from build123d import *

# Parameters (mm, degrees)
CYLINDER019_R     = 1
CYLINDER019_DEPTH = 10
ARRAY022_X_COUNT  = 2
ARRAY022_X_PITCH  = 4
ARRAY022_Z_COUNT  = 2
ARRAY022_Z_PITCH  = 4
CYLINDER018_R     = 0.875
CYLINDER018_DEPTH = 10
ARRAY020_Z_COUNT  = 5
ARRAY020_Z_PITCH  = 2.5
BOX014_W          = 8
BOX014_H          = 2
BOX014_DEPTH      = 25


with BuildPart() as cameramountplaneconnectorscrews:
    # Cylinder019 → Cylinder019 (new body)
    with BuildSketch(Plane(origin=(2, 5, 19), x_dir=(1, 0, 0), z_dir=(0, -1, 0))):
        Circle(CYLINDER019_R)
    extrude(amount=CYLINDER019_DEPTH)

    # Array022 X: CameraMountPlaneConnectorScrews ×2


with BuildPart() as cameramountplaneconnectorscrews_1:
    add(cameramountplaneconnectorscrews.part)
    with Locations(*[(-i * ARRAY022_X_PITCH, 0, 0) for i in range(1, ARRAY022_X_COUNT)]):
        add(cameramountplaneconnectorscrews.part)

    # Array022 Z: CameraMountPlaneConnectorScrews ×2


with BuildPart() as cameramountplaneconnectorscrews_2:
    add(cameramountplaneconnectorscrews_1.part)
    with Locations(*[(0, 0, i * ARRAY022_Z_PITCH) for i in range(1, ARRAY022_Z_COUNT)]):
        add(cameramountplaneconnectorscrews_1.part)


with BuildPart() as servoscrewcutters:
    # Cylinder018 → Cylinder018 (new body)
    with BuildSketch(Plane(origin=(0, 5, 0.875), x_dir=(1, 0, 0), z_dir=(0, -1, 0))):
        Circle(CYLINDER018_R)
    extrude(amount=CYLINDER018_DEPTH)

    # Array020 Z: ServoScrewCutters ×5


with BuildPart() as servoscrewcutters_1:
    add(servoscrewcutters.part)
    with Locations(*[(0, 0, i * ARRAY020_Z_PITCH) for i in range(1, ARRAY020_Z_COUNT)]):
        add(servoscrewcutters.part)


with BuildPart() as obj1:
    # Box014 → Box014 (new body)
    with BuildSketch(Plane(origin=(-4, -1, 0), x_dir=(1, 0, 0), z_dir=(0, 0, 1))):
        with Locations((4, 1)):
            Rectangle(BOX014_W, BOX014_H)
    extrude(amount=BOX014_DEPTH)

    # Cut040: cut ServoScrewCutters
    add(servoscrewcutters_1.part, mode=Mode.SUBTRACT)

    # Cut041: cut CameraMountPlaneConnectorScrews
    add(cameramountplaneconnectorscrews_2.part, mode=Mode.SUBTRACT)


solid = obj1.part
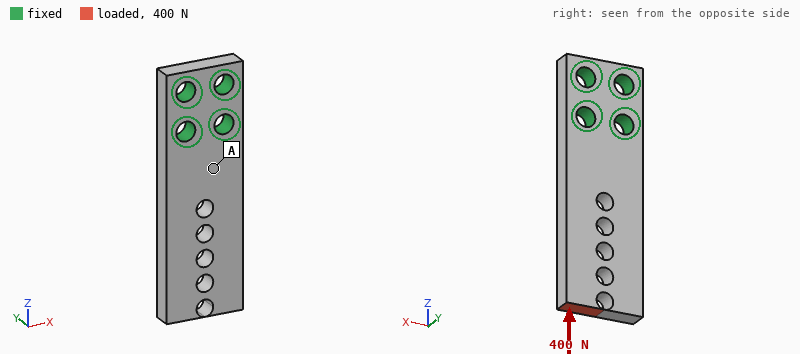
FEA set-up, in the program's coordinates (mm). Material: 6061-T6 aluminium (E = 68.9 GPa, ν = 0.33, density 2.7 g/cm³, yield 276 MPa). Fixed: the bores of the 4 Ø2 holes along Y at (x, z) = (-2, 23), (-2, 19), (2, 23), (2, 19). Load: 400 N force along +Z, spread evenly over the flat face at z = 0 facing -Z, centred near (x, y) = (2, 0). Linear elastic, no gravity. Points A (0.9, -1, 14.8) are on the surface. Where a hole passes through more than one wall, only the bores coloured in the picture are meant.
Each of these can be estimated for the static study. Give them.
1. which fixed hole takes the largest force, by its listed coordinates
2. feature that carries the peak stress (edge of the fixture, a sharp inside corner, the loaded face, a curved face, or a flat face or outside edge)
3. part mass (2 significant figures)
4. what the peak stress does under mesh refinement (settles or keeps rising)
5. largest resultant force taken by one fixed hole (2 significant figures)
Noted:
(2, 19)
a sharp inside corner
0.95 g
keeps rising
340 N
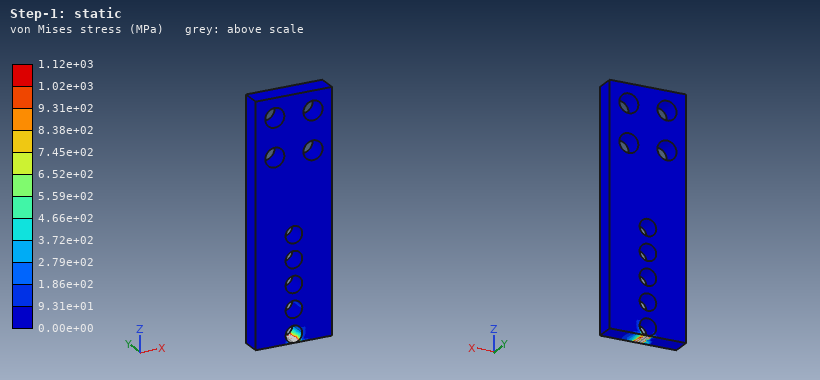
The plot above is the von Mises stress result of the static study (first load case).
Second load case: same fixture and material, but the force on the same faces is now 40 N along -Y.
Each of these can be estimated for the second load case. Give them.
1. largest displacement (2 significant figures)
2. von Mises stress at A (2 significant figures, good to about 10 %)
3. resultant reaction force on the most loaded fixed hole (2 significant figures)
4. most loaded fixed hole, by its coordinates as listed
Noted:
0.26 mm
110 MPa
39 N
(2, 19)
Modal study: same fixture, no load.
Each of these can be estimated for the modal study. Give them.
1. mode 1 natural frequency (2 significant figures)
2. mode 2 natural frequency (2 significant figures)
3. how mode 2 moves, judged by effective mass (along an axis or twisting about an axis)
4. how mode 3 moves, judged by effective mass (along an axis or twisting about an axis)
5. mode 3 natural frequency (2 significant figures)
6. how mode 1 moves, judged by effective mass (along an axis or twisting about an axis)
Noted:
5100 Hz
17 kHz
along X
twisting about Z
19 kHz
along Y
